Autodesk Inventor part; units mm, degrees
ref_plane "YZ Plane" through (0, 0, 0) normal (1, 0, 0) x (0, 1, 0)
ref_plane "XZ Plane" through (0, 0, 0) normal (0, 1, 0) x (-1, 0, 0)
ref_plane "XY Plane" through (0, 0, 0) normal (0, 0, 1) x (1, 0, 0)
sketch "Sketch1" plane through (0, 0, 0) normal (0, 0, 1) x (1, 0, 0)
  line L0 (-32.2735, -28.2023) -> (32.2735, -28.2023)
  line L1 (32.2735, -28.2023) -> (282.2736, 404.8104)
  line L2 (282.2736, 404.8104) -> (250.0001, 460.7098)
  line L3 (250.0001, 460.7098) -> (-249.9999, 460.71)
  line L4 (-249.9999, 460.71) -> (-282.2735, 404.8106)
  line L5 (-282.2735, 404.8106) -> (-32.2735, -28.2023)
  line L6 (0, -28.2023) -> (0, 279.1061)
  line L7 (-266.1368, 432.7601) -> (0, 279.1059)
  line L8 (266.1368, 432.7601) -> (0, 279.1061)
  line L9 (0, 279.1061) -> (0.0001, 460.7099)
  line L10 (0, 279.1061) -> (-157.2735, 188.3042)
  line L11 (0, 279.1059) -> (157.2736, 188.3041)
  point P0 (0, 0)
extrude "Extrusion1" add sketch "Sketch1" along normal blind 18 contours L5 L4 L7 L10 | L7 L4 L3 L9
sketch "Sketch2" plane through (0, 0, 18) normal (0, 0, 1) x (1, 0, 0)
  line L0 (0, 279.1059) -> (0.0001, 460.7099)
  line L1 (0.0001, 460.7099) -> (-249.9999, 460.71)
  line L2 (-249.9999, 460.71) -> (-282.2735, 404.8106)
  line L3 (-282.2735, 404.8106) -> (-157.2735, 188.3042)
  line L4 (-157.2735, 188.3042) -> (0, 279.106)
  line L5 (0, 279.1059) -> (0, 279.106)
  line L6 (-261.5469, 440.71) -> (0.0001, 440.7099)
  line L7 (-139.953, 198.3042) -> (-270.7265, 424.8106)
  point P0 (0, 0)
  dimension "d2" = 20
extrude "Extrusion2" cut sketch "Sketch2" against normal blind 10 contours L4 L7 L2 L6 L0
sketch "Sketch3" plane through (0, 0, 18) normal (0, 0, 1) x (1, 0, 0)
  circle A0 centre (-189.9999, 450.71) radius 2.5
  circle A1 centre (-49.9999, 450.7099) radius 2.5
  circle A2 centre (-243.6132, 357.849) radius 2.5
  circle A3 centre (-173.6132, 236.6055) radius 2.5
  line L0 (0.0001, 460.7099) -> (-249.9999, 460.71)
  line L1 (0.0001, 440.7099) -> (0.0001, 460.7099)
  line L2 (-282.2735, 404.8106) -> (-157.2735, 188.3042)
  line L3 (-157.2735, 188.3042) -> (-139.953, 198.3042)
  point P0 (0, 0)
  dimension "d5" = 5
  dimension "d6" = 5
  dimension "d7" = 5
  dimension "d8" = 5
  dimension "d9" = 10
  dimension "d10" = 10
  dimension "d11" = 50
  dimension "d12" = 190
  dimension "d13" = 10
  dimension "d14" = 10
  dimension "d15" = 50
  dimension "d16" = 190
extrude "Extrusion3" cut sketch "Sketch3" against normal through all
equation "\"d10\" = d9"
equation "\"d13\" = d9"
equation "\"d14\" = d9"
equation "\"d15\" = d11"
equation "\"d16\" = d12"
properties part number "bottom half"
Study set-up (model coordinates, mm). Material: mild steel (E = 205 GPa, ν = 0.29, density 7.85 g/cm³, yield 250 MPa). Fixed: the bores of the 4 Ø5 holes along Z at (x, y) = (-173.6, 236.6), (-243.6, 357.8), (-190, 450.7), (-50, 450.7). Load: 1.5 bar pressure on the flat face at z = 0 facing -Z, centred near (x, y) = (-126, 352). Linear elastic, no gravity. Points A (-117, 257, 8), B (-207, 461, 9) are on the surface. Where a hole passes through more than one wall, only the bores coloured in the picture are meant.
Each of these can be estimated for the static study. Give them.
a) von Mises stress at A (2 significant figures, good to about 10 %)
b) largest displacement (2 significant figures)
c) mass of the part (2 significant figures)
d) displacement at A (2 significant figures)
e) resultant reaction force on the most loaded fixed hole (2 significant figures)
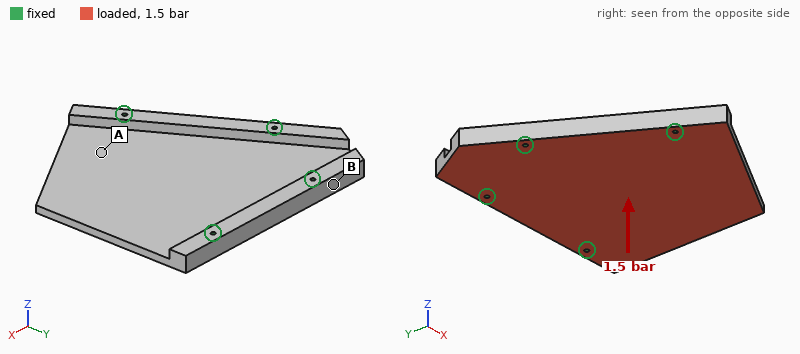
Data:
25 MPa
0.59 mm
4.3 kg
0.14 mm
3.6 kN
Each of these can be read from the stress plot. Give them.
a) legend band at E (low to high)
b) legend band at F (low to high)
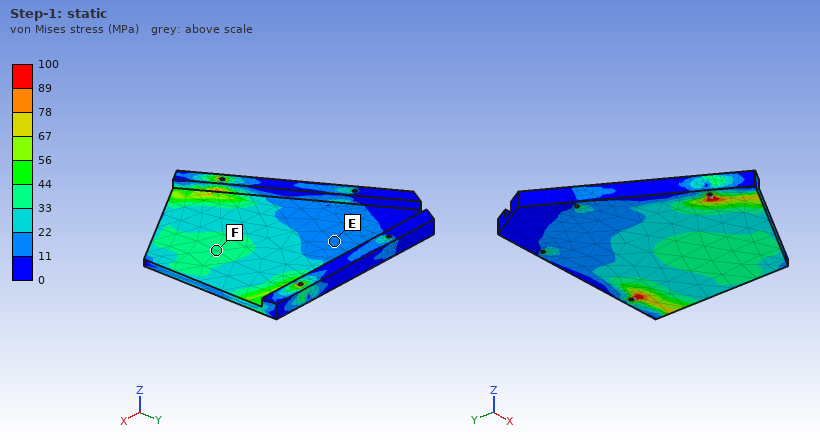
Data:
11 to 22 MPa
33 to 44 MPa
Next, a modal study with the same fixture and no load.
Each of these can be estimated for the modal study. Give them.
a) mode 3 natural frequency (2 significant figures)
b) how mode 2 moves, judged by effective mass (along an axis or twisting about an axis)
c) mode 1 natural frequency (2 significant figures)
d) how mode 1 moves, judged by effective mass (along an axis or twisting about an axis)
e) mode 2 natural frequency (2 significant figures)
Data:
1300 Hz
along Z
460 Hz
along Z
1300 Hz
